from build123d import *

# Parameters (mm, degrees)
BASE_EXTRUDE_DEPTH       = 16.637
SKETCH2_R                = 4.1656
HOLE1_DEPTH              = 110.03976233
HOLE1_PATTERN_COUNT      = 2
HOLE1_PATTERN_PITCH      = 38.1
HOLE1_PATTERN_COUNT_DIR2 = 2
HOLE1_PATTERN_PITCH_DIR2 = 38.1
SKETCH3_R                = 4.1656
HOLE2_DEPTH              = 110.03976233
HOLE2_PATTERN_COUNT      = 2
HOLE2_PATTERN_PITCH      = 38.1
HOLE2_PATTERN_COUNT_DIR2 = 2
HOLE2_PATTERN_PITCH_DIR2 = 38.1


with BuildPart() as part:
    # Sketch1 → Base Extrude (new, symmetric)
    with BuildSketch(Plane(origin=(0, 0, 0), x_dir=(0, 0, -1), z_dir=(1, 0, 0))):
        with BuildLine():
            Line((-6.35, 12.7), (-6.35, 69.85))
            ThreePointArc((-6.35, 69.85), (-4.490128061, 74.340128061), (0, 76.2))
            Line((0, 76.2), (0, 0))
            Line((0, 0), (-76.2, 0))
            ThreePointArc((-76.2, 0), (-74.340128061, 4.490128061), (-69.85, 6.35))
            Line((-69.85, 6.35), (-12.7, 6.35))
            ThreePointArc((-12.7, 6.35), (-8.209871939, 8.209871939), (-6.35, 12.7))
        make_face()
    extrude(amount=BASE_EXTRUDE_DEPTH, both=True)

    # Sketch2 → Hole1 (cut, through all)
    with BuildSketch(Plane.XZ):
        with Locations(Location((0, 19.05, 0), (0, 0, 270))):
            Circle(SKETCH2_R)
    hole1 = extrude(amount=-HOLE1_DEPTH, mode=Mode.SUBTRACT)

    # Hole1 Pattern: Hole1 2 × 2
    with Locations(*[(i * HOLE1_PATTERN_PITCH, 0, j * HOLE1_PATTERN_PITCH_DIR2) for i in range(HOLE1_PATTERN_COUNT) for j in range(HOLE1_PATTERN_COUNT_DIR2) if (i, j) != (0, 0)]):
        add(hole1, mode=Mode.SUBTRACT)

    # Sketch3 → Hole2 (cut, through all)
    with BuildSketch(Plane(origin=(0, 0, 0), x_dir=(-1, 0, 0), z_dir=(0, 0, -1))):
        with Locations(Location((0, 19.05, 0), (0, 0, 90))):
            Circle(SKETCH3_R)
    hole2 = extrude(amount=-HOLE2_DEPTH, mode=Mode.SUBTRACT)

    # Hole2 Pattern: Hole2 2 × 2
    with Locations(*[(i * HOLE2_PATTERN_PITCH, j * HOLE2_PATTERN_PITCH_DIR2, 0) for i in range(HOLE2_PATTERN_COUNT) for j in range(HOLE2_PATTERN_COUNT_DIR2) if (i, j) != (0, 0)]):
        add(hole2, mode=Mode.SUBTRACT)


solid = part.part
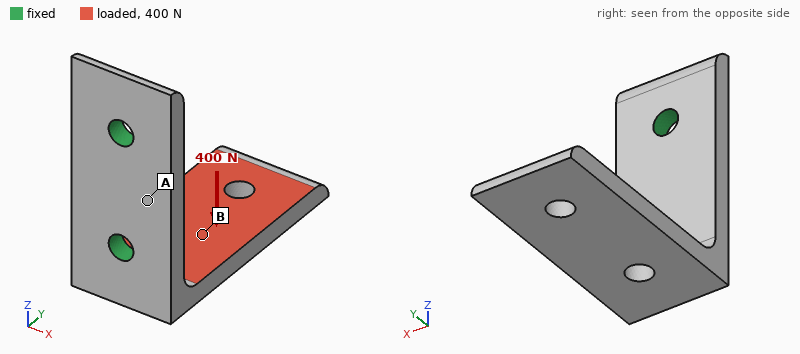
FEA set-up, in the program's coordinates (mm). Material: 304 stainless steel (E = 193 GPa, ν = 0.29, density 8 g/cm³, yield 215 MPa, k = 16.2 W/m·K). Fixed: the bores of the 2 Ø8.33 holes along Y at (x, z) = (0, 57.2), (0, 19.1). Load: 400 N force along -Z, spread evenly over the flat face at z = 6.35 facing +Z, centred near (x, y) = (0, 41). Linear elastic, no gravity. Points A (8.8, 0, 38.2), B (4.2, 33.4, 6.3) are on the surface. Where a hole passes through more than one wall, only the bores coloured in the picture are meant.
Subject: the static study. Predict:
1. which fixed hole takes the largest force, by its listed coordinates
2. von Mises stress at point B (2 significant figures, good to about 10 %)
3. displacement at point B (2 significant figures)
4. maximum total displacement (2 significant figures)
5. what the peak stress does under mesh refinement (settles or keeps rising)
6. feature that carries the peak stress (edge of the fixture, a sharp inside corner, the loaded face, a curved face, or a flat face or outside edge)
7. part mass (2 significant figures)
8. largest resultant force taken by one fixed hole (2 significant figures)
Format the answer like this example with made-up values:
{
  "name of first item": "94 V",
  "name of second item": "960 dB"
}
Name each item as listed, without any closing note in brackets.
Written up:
{
  "which fixed hole takes the largest force, by its listed coordinates": "(0, 19.1)",
  "von Mises stress at point B": "20 MPa",
  "displacement at point B": "0.064 mm",
  "maximum total displacement": "0.21 mm",
  "what the peak stress does under mesh refinement": "keeps rising",
  "feature that carries the peak stress": "edge of the fixture",
  "part mass": "230 g",
  "largest resultant force taken by one fixed hole": "380 N"
}
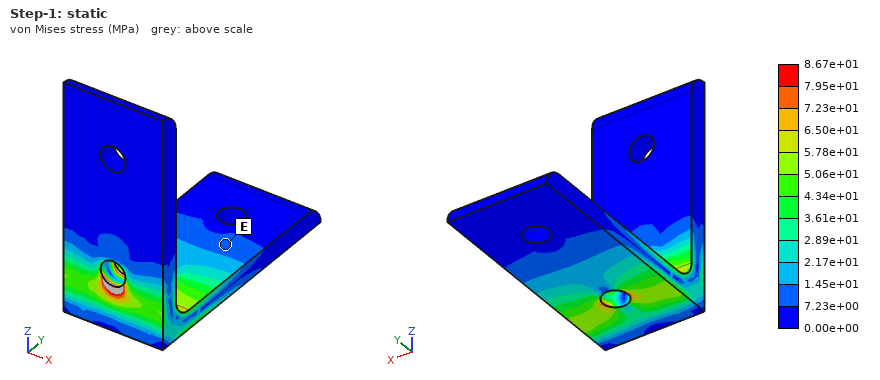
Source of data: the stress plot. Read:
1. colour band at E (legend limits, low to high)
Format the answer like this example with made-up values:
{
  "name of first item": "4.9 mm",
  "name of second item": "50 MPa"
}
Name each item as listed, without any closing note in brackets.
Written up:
{
  "colour band at E": "7.23e+00 to 1.45e+01 MPa"
}
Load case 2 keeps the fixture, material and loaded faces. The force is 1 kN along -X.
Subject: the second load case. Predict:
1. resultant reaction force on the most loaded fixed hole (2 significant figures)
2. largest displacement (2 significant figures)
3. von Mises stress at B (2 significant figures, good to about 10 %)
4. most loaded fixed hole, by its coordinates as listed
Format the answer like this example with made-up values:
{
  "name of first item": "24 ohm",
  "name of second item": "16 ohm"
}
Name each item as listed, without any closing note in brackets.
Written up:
{
  "resultant reaction force on the most loaded fixed hole": "1.2 kN",
  "largest displacement": "0.14 mm",
  "von Mises stress at B": "20 MPa",
  "most loaded fixed hole, by its coordinates as listed": "(0, 19.1)"
}
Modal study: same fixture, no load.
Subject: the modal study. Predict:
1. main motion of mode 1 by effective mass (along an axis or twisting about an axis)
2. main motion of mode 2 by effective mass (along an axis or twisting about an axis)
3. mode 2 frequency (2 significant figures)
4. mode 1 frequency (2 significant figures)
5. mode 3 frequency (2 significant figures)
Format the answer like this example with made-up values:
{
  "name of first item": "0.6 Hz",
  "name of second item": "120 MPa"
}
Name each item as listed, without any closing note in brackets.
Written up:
{
  "main motion of mode 1 by effective mass": "along Z",
  "main motion of mode 2 by effective mass": "along X",
  "mode 2 frequency": "1600 Hz",
  "mode 1 frequency": "820 Hz",
  "mode 3 frequency": "4000 Hz"
}
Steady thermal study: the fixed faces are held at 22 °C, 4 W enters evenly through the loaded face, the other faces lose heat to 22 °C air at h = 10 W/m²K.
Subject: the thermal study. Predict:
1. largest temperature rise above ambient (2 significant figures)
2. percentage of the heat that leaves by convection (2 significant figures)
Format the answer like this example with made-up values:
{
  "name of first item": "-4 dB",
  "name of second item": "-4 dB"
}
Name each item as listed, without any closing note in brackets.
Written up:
{
  "largest temperature rise above ambient": "40 K",
  "percentage of the heat that leaves by convection": "34 %"
}
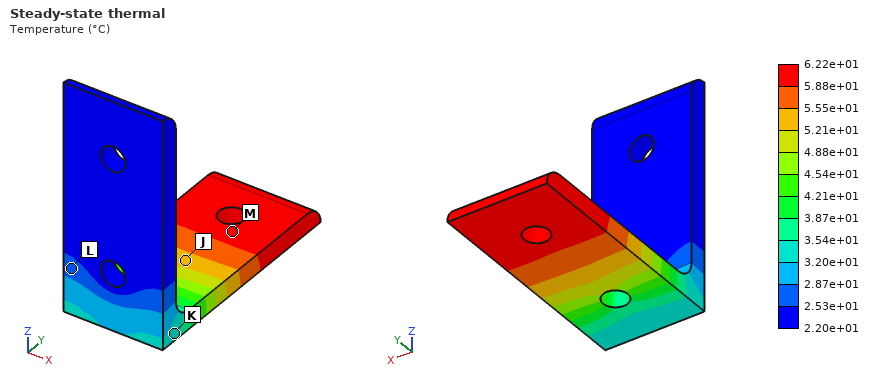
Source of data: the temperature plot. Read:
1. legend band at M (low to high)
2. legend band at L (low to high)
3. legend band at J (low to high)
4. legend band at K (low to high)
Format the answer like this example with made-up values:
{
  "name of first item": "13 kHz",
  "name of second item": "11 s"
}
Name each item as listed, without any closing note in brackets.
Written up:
{
  "legend band at M": "5.88e+01 to 6.22e+01 °C",
  "legend band at L": "2.53e+01 to 2.87e+01 °C",
  "legend band at J": "5.21e+01 to 5.55e+01 °C",
  "legend band at K": "3.20e+01 to 3.54e+01 °C"
}
